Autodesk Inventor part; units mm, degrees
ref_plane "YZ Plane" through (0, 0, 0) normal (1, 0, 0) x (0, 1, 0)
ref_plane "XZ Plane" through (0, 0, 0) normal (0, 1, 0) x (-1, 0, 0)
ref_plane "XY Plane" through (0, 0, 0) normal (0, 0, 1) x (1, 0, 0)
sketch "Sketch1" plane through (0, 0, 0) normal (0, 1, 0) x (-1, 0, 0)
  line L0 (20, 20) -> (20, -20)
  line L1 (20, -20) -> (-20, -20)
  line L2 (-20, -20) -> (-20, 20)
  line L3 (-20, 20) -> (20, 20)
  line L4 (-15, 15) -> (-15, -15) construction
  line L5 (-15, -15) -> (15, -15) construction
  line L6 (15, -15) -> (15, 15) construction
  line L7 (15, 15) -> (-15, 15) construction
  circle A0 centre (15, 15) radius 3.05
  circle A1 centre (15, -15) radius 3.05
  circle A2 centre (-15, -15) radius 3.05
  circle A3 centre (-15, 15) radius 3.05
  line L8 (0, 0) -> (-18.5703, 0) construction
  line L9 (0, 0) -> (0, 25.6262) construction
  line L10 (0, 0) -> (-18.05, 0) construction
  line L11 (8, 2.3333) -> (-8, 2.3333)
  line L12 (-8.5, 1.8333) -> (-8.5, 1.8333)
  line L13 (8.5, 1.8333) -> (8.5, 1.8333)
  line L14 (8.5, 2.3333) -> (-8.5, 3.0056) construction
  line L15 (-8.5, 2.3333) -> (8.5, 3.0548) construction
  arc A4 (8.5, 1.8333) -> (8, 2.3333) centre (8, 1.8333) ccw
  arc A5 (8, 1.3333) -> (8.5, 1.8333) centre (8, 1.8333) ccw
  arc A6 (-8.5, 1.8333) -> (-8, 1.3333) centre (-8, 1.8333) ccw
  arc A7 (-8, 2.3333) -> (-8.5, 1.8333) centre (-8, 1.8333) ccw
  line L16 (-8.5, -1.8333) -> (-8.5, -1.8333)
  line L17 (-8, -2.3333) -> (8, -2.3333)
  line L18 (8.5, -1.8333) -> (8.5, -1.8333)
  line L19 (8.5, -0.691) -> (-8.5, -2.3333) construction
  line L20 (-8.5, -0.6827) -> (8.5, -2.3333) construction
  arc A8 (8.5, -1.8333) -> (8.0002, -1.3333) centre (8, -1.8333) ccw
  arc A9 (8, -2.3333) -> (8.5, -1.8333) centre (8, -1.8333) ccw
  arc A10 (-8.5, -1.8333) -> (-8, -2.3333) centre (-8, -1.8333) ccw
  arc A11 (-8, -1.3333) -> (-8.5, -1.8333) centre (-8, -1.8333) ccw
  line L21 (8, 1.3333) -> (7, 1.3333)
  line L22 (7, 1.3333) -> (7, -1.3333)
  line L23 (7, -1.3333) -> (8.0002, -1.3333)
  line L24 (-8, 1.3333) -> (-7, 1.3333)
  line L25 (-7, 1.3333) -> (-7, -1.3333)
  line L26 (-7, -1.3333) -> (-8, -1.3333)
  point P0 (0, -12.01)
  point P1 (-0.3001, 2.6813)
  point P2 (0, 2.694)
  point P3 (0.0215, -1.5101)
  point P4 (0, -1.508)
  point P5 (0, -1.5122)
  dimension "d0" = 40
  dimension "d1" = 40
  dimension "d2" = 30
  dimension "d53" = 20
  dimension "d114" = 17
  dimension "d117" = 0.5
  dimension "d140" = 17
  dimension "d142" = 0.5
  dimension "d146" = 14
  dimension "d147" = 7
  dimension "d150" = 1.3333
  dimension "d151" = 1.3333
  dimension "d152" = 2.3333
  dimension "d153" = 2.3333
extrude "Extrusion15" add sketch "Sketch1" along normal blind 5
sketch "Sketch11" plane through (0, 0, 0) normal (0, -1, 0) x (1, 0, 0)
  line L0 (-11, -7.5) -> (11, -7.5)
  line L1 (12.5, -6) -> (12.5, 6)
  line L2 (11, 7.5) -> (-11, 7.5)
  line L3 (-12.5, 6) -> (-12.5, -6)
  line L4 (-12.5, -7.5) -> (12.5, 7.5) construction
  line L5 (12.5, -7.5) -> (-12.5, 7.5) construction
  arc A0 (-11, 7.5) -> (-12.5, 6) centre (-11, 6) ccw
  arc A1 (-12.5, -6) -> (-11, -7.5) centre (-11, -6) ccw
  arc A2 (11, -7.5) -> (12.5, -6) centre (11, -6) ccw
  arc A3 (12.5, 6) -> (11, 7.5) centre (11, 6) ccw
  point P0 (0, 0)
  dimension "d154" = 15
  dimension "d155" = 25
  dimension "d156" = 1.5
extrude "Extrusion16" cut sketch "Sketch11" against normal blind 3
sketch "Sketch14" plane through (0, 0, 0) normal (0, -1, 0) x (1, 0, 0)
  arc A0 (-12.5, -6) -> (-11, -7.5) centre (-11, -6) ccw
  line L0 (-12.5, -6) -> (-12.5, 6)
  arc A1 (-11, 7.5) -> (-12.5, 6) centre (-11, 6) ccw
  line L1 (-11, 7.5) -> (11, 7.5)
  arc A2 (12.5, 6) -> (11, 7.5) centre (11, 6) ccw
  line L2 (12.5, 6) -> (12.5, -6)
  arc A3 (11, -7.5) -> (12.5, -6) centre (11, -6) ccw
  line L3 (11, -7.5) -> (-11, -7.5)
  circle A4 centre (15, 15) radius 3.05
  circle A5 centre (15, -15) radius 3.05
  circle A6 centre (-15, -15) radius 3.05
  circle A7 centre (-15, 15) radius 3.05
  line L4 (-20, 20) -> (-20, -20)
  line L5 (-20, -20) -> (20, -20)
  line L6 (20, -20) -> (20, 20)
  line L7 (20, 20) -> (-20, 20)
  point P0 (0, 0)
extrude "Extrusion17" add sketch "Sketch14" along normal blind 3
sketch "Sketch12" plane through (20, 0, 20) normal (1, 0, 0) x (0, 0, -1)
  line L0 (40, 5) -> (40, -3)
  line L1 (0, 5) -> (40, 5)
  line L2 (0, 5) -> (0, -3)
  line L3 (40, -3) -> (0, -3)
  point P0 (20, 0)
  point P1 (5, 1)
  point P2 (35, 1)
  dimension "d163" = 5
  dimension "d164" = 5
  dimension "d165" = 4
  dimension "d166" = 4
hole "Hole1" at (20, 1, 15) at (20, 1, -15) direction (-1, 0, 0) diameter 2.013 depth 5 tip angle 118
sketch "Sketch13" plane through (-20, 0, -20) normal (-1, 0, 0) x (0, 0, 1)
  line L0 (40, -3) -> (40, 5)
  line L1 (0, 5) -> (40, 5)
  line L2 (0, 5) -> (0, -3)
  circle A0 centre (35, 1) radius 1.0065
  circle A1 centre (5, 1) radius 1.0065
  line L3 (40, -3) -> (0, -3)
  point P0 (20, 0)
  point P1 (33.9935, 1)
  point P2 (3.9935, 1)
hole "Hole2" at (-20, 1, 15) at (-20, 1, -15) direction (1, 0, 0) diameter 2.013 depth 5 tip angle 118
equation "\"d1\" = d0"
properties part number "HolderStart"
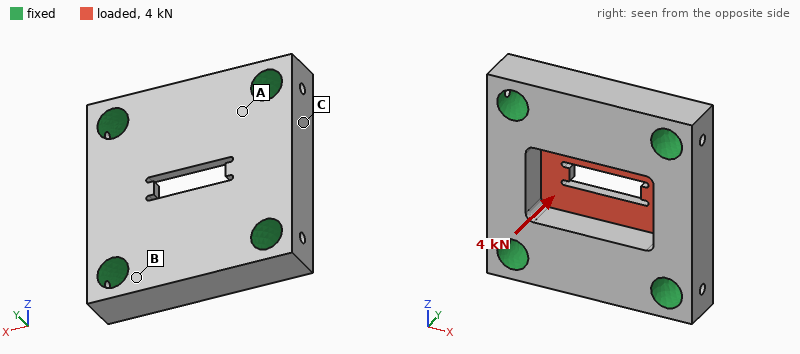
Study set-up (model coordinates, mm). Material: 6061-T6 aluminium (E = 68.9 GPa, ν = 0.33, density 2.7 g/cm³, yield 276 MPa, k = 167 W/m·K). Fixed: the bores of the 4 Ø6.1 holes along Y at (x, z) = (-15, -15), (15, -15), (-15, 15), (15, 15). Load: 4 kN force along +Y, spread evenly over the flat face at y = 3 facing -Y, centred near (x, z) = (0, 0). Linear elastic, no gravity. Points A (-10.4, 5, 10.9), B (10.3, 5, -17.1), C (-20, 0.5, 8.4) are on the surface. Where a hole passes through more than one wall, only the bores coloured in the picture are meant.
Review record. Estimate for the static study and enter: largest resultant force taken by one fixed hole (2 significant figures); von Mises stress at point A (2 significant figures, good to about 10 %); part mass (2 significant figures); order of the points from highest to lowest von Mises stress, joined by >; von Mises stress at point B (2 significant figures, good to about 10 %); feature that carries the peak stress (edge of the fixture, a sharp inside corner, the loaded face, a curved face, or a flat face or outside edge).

1.0 kN
47 MPa
26 g
A > B > C
30 MPa
a curved face
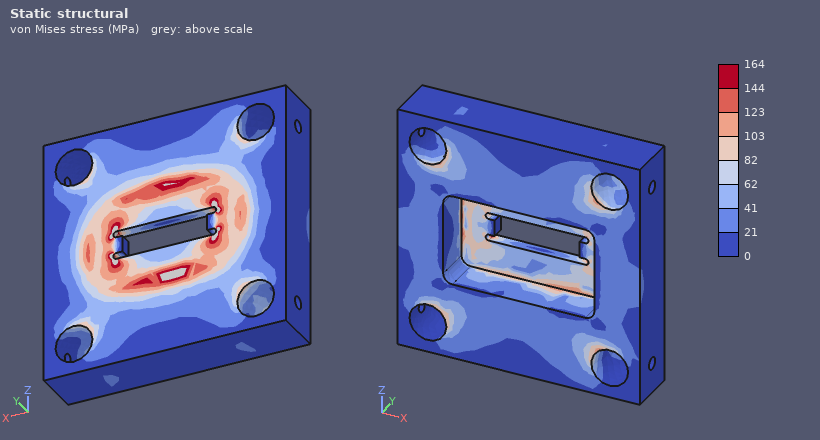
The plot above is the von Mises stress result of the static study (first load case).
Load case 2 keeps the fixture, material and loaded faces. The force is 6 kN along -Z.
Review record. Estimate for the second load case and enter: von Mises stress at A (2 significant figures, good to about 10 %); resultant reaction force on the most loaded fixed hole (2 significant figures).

49 MPa
1.6 kN
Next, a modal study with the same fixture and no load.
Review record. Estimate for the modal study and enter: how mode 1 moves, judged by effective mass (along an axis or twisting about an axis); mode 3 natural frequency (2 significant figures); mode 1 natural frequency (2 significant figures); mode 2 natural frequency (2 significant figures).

along Y
42 kHz
32 kHz
35 kHz
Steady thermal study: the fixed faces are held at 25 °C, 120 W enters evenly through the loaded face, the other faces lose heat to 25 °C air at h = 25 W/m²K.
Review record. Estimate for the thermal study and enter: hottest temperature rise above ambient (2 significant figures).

37 K
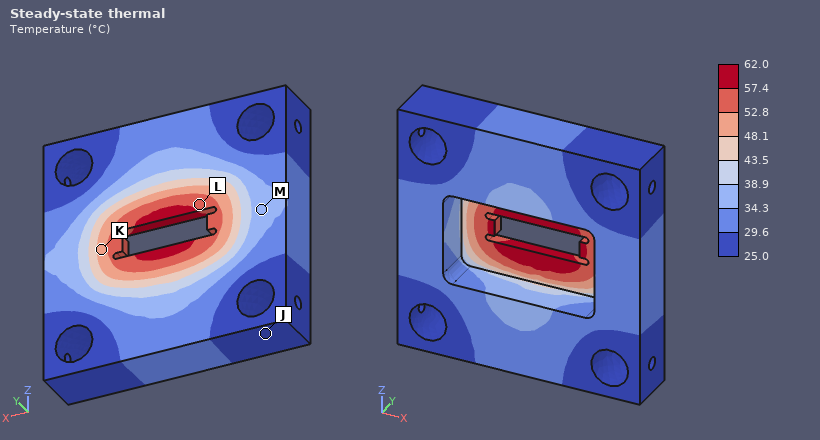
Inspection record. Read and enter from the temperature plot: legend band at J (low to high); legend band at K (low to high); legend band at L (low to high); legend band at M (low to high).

25.0 to 29.6 °C
48.1 to 52.8 °C
52.8 to 57.4 °C
34.3 to 38.9 °C
